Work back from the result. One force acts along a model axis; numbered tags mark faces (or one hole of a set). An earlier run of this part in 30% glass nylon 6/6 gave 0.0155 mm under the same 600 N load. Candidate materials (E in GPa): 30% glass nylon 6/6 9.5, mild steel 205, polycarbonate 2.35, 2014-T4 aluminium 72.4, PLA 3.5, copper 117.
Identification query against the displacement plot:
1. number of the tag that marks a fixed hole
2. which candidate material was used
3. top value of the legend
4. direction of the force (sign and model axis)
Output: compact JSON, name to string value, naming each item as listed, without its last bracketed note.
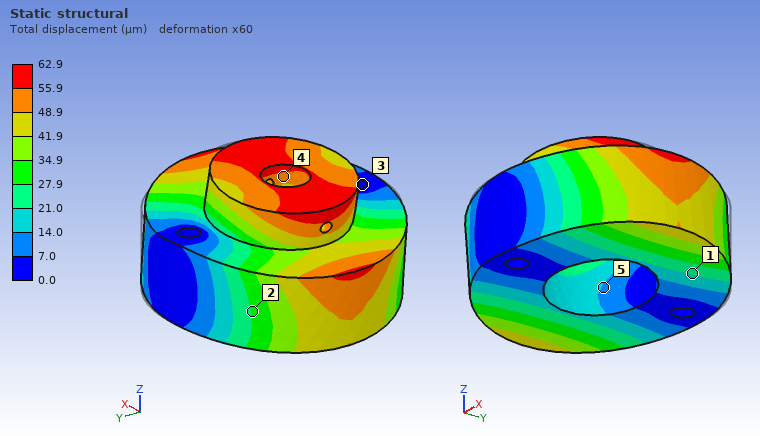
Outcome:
{"number of the tag that marks a fixed hole": "3", "which candidate material was used": "polycarbonate", "top value of the legend": "62.9 µm", "direction of the force": "-X"}
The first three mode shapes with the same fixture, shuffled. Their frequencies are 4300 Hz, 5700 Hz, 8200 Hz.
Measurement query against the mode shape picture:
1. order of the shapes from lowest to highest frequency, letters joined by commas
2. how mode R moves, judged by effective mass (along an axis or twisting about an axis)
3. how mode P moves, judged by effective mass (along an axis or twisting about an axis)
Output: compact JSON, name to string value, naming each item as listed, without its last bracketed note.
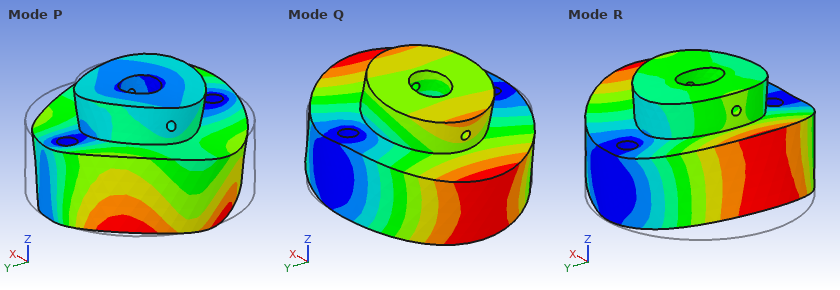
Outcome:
{"order of the shapes from lowest to highest frequency, letters joined by commas": "Q, R, P", "how mode R moves, judged by effective mass": "along Z", "how mode P moves, judged by effective mass": "twisting about Z"}
